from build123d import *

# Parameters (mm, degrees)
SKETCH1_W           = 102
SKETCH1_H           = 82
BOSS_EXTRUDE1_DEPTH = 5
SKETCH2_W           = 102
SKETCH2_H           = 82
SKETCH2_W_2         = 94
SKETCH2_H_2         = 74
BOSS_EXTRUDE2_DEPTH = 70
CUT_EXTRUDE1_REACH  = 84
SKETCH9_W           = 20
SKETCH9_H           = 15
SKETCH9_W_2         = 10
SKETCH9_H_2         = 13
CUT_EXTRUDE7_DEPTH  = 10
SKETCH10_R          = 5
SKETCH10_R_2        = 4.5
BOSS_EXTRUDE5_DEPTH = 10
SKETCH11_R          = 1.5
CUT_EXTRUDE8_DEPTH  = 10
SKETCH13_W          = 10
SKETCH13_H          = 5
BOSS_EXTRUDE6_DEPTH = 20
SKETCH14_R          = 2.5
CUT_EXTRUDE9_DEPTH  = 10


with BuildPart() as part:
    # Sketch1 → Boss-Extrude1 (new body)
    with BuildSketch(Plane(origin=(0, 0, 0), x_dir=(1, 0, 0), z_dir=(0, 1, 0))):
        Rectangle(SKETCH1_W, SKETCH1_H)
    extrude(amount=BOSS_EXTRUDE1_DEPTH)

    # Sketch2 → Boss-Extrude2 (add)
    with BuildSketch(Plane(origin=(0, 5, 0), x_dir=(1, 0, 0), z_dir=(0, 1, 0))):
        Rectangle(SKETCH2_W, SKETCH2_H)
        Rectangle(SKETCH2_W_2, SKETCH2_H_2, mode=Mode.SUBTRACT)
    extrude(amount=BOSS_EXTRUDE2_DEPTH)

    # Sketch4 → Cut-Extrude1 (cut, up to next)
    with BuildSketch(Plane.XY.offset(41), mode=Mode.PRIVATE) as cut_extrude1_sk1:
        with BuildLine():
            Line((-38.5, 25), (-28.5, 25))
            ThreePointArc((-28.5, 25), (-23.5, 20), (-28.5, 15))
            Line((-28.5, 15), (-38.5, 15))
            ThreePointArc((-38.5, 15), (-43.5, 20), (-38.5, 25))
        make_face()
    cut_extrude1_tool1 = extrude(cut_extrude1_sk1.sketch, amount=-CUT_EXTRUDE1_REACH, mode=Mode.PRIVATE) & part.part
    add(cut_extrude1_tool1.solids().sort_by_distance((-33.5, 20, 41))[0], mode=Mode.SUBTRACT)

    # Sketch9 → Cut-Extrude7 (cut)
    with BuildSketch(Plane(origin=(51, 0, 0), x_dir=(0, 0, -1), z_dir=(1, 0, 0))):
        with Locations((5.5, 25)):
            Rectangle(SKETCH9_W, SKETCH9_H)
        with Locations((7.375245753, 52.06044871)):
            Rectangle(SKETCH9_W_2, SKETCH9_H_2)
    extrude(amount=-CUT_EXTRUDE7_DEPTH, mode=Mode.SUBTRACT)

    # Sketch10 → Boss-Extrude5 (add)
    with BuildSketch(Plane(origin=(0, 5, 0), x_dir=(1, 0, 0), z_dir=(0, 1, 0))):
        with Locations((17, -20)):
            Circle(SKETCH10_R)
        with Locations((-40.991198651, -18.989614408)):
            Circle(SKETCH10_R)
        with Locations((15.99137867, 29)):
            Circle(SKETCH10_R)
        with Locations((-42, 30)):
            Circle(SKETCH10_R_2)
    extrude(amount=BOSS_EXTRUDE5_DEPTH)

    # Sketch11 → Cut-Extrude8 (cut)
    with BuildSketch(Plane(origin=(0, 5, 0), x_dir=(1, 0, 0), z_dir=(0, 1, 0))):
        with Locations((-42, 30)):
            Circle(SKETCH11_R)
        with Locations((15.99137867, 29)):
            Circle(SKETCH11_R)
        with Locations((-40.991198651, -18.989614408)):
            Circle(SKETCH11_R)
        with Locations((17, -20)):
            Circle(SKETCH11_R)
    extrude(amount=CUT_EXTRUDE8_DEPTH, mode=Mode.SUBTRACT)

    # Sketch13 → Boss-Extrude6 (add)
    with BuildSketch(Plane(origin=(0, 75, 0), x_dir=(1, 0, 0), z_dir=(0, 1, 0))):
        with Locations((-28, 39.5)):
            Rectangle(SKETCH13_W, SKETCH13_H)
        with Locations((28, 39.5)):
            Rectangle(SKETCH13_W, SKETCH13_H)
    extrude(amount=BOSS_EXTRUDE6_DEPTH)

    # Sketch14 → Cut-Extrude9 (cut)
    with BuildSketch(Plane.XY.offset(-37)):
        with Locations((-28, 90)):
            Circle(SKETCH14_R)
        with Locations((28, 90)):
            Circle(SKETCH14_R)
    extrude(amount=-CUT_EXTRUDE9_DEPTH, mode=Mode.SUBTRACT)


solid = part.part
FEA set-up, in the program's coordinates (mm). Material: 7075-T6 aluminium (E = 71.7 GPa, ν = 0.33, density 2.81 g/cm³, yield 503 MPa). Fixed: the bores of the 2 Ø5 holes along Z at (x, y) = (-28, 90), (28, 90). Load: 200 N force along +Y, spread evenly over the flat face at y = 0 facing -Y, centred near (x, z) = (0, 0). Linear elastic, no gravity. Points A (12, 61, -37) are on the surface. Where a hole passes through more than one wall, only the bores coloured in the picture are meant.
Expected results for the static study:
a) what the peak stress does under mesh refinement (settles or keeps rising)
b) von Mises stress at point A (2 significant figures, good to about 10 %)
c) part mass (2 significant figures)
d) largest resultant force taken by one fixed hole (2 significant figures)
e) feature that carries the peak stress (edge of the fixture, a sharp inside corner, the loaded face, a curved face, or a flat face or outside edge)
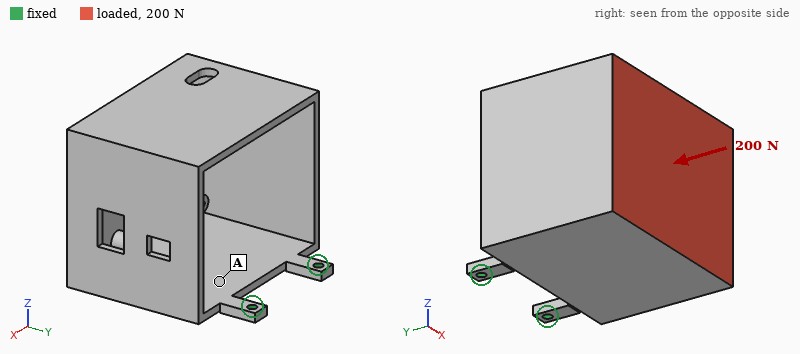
keeps rising
15 MPa
400 g
100 N
a sharp inside corner
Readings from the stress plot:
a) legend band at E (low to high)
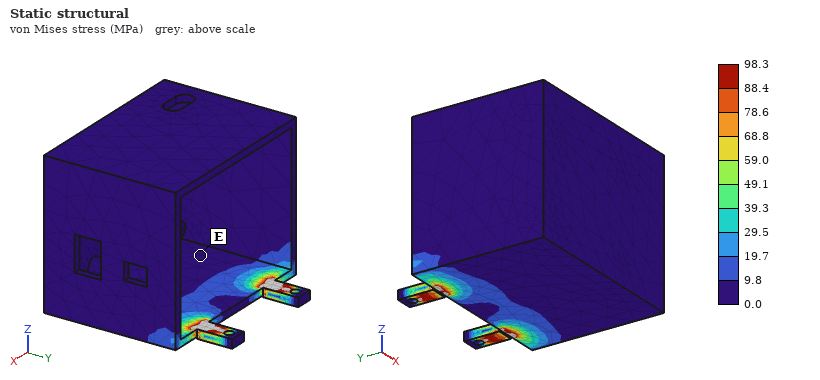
0.0 to 9.8 MPa
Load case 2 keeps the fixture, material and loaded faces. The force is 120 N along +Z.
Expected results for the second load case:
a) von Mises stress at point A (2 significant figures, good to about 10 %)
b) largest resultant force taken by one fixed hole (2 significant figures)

15 MPa
61 N
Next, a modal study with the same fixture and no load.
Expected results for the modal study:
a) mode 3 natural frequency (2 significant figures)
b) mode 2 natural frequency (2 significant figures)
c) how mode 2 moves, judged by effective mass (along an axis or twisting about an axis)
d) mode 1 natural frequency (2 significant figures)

650 Hz
210 Hz
along X
80 Hz
